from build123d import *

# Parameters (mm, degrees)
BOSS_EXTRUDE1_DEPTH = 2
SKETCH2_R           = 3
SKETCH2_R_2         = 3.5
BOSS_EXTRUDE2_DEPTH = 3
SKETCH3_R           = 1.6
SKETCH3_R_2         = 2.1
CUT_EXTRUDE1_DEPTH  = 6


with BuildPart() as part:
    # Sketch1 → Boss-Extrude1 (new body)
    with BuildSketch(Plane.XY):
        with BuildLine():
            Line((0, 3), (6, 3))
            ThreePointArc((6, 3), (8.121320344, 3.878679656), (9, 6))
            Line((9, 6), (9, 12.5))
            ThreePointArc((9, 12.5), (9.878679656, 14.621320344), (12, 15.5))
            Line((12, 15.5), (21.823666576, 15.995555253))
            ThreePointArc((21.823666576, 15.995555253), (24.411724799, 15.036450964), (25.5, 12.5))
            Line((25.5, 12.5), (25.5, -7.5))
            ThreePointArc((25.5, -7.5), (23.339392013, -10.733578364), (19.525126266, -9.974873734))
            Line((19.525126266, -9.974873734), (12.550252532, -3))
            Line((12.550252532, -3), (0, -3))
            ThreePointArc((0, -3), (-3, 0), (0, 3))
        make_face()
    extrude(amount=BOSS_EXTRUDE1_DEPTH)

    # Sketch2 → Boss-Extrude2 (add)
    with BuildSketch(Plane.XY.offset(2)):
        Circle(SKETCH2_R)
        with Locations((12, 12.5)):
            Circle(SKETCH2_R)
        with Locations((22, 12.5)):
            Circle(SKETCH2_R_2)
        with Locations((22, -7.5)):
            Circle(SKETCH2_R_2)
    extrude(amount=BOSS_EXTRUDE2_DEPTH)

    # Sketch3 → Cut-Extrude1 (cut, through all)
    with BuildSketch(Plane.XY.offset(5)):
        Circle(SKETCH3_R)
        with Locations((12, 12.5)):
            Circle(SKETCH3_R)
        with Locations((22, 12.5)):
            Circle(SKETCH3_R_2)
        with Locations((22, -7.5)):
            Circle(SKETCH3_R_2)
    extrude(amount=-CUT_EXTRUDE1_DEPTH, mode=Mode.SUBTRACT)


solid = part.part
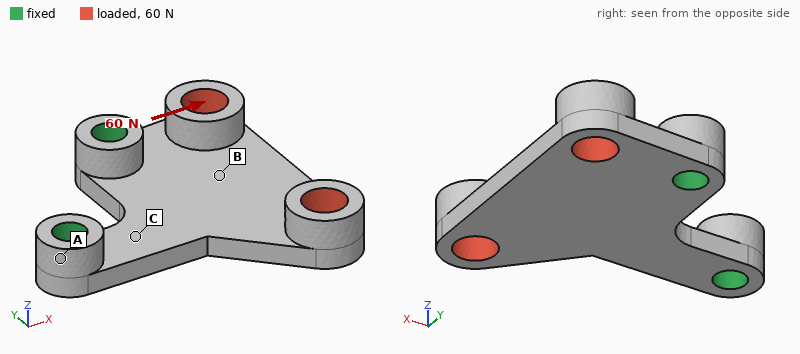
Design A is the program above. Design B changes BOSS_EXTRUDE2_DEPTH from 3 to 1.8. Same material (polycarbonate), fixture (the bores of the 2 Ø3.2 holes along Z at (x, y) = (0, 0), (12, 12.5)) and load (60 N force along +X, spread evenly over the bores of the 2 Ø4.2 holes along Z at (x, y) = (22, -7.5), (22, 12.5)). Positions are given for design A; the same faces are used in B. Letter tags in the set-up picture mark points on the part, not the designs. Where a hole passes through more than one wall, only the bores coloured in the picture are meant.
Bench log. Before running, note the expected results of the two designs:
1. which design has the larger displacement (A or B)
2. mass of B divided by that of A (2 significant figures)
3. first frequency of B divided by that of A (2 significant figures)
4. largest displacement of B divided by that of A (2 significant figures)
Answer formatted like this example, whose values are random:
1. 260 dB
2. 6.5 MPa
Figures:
1. A
2. 0.90
3. 1.1
4. 0.61
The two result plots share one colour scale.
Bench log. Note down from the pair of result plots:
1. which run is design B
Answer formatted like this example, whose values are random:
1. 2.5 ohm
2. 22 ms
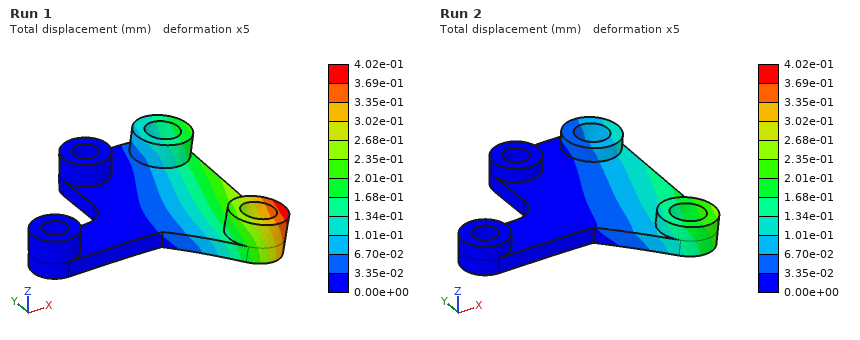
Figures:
1. Run 2
